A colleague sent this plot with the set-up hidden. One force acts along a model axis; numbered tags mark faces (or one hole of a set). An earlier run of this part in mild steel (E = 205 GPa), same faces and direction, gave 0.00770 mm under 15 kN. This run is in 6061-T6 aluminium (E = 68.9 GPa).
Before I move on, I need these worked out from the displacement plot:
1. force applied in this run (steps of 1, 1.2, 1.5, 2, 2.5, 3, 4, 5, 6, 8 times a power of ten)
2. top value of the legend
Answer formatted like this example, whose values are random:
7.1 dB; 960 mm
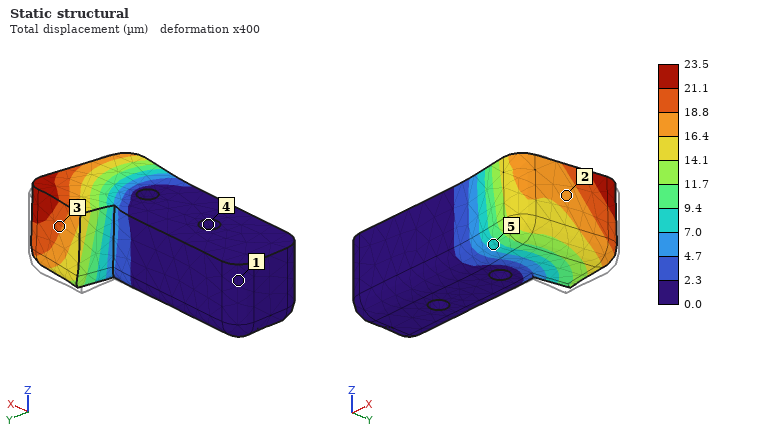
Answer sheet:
15 kN; 23.5 µm
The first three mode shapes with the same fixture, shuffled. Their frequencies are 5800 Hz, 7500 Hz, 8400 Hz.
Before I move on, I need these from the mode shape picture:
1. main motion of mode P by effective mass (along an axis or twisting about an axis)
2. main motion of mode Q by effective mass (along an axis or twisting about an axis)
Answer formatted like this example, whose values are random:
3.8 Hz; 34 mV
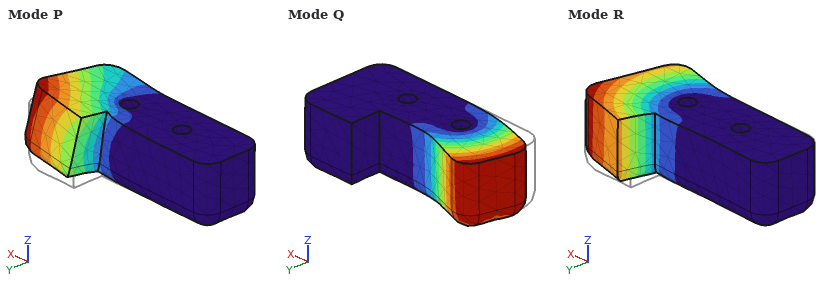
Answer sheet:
along Z; along Y
